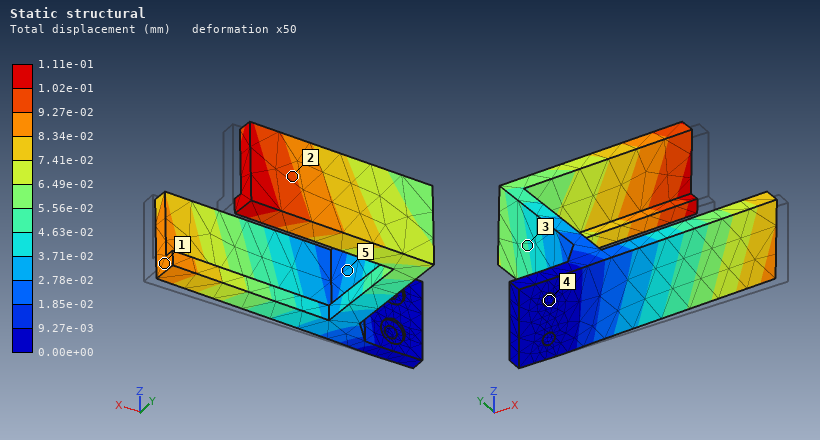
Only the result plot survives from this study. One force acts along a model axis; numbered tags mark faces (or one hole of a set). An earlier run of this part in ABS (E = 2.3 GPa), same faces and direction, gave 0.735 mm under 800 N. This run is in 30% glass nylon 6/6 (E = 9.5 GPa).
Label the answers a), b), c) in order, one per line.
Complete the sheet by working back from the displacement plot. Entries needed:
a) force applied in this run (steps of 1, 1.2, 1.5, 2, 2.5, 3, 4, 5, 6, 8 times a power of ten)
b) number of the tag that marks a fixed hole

a) 500 N
b) 4
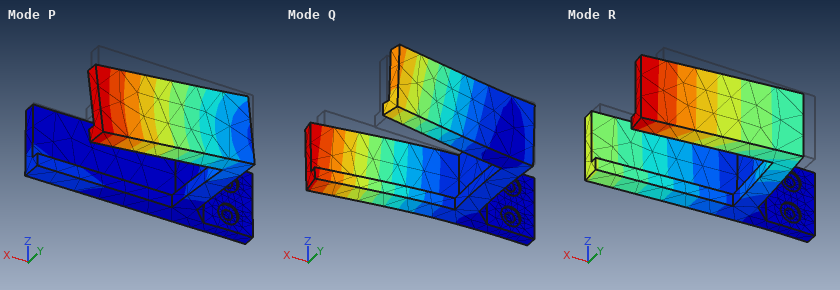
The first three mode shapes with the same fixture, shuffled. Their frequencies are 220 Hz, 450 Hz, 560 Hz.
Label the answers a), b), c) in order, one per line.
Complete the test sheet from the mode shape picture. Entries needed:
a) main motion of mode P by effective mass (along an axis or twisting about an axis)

a) along Z
